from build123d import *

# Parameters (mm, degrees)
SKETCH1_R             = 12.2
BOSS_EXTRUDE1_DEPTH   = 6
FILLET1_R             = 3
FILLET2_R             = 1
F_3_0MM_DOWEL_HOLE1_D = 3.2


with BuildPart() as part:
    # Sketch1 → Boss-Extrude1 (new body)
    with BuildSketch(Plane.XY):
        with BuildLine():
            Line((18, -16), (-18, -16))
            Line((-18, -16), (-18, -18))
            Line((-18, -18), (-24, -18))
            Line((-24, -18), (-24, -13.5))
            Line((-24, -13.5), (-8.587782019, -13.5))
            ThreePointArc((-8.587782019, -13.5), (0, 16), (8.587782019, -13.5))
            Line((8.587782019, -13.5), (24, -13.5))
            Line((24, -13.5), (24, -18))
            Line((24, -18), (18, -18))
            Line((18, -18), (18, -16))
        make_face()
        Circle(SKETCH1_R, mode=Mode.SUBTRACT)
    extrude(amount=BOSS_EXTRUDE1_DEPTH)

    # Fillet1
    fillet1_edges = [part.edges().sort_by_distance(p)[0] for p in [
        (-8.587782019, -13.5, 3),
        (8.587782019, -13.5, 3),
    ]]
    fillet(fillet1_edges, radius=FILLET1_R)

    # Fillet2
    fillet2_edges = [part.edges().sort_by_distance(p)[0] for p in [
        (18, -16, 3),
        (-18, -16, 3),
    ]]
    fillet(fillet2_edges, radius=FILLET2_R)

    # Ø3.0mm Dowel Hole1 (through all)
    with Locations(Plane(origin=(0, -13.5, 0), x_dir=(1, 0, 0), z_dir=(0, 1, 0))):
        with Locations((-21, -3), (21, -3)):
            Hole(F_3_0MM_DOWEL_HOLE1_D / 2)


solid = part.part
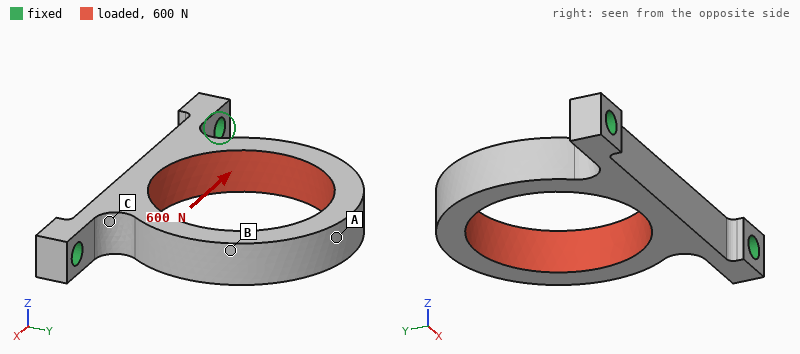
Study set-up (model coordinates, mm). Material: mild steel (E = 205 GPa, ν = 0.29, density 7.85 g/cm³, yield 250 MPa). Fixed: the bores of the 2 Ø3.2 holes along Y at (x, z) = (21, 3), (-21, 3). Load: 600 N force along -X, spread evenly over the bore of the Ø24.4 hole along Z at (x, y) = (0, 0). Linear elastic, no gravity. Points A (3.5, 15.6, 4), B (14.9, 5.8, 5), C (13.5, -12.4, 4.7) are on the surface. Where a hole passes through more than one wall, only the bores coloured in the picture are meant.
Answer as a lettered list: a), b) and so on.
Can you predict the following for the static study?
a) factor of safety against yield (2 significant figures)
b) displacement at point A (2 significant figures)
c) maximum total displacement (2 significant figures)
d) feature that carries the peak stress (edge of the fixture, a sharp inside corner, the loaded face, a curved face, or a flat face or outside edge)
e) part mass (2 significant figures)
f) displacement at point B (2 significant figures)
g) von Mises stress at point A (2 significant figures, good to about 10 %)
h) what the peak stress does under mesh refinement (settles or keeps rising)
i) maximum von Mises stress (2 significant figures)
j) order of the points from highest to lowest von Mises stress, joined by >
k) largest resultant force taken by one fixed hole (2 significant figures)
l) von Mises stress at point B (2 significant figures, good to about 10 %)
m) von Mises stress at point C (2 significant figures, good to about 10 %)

a) 1.9
b) 40 µm
c) 40 µm
d) a curved face
e) 22 g
f) 34 µm
g) 19 MPa
h) settles
i) 130 MPa
j) C > B > A
k) 400 N
l) 42 MPa
m) 95 MPa
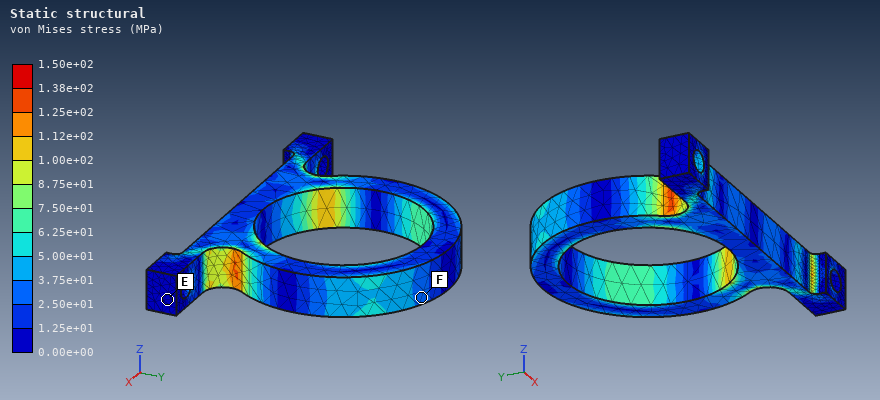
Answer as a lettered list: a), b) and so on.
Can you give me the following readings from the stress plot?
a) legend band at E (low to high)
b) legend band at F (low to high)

a) 0.00e+00 to 1.25e+01 MPa
b) 2.50e+01 to 3.75e+01 MPa
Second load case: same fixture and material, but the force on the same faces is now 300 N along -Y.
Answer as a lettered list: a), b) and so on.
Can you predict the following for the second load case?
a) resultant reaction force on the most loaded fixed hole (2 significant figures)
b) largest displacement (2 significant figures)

a) 190 N
b) 5.5 µm
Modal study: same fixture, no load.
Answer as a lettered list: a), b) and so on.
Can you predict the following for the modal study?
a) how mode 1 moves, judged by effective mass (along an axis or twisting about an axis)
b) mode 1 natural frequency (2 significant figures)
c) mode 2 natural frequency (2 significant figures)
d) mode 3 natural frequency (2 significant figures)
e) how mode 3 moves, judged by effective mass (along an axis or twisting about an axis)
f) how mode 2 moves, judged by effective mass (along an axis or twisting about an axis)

a) along Z
b) 1900 Hz
c) 5300 Hz
d) 7100 Hz
e) twisting about Y
f) along X
